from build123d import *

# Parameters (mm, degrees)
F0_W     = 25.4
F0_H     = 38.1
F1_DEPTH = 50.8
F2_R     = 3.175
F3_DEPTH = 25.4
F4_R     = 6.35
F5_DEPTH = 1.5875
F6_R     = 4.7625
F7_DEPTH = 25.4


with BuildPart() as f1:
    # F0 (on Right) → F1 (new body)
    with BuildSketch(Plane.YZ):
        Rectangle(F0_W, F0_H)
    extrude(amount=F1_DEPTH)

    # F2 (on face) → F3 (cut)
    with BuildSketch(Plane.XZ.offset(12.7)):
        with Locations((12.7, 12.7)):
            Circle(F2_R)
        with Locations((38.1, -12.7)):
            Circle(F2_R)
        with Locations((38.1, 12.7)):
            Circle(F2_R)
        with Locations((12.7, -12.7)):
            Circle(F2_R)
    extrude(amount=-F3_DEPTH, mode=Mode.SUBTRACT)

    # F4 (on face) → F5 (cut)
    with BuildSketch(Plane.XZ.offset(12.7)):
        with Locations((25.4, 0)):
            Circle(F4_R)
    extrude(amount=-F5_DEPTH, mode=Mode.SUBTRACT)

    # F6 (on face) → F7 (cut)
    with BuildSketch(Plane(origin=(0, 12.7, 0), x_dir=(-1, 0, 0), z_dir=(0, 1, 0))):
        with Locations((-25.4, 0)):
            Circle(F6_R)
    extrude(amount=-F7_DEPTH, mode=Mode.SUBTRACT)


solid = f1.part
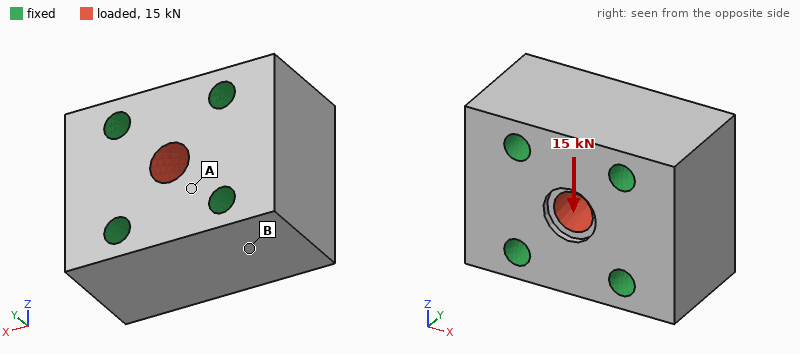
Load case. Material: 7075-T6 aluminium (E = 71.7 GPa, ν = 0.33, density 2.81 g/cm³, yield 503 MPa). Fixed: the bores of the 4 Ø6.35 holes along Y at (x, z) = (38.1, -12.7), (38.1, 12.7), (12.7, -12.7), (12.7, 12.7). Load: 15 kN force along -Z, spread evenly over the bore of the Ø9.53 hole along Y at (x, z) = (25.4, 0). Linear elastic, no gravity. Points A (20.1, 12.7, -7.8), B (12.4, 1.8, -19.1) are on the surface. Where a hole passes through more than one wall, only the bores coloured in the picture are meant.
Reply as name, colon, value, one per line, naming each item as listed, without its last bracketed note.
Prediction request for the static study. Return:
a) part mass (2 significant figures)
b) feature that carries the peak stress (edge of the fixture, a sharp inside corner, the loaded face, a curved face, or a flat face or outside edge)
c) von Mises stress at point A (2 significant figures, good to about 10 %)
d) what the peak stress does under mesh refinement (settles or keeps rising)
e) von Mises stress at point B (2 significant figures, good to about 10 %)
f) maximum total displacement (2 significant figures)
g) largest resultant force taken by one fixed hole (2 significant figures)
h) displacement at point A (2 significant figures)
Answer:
part mass: 120 g
feature that carries the peak stress: edge of the fixture
von Mises stress at point A: 18 MPa
what the peak stress does under mesh refinement: keeps rising
von Mises stress at point B: 5.3 MPa
maximum total displacement: 4.3 µm
largest resultant force taken by one fixed hole: 4.1 kN
displacement at point A: 2.2 µm
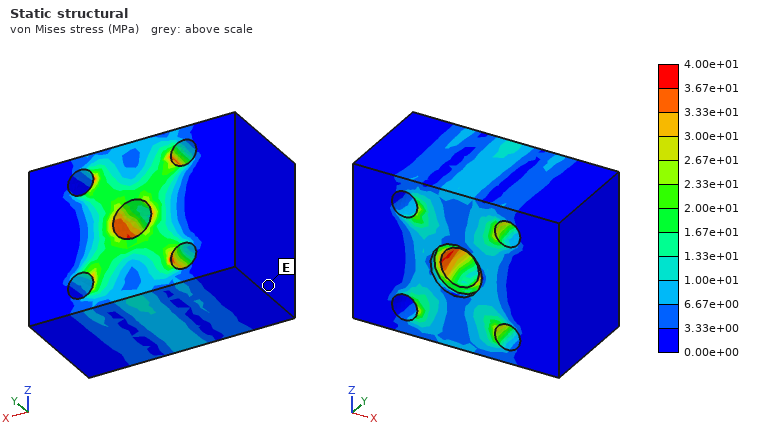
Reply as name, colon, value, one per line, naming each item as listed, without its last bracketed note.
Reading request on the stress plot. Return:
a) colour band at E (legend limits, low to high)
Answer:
colour band at E: 0.00e+00 to 3.33e+00 MPa
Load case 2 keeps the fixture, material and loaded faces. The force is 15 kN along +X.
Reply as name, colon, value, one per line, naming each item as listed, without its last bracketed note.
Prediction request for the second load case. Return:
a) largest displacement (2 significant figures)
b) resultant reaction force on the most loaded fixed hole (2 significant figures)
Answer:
largest displacement: 3.9 µm
resultant reaction force on the most loaded fixed hole: 4.0 kN
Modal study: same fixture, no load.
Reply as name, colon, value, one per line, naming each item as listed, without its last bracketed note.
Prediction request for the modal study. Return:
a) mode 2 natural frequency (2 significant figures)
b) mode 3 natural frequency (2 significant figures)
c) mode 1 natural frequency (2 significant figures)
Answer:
mode 2 natural frequency: 49 kHz
mode 3 natural frequency: 57 kHz
mode 1 natural frequency: 49 kHz
